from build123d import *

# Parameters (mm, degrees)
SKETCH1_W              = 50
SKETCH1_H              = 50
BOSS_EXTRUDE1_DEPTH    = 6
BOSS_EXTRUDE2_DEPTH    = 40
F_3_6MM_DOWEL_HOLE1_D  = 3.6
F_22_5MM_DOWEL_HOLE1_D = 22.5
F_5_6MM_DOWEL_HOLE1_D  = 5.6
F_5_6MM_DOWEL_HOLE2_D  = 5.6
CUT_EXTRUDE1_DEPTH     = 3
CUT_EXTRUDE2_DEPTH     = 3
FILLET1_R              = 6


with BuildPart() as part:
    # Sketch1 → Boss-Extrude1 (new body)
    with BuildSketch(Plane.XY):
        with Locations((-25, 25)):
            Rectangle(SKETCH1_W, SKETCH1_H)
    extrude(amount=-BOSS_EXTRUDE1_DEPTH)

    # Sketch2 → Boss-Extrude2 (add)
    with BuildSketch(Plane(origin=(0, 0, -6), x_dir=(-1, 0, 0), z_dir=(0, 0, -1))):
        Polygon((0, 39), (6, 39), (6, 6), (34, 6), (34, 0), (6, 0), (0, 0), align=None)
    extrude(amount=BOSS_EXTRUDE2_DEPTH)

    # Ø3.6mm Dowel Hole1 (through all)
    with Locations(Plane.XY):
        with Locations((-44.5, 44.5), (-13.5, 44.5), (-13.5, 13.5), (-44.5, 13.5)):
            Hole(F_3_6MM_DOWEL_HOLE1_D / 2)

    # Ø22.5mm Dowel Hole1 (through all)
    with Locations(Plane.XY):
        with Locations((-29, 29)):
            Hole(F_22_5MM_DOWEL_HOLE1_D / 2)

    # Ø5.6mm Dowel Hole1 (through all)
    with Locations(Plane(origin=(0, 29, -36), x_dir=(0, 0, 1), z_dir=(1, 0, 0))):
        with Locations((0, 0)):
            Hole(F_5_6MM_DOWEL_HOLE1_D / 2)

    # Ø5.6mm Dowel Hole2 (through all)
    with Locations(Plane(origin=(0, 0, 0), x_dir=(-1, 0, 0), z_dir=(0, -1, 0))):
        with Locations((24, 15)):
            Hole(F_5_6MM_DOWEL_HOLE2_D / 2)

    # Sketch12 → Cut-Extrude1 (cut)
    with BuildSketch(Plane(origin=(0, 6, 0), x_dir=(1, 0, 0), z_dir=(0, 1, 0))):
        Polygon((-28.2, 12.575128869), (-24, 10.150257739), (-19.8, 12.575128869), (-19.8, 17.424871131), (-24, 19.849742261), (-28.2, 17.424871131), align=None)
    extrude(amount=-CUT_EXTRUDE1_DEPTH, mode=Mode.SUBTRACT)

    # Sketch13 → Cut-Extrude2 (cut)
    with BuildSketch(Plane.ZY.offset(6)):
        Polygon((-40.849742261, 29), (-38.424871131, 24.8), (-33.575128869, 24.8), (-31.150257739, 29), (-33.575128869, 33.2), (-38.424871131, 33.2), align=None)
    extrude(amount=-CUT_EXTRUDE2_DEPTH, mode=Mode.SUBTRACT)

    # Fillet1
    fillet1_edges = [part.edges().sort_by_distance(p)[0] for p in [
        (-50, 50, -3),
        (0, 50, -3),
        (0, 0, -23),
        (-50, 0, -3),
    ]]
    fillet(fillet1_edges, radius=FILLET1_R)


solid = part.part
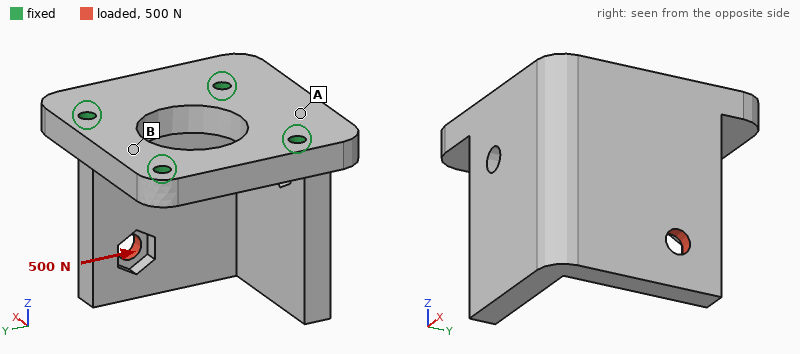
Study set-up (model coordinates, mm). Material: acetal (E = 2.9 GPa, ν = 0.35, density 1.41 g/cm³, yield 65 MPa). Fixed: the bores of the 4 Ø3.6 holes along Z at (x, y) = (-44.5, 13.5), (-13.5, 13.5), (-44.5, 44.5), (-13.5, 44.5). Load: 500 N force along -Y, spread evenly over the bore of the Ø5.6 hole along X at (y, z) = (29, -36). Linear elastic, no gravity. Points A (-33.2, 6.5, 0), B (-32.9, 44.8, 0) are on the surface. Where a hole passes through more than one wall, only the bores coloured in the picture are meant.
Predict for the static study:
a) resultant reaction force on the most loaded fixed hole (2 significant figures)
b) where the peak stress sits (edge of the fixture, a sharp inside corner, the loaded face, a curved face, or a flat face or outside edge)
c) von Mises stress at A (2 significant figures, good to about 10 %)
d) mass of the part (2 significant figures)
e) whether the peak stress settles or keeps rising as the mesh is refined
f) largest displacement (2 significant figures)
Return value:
590 N
edge of the fixture
7.2 MPa
39 g
keeps rising
0.84 mm
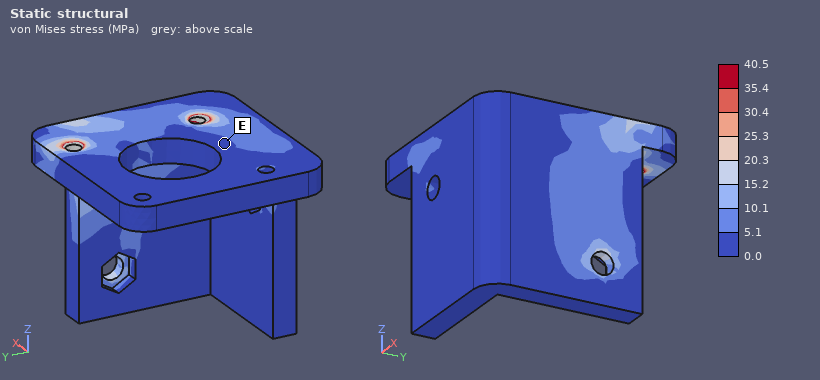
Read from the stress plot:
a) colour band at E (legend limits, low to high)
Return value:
0.0 to 5.1 MPa
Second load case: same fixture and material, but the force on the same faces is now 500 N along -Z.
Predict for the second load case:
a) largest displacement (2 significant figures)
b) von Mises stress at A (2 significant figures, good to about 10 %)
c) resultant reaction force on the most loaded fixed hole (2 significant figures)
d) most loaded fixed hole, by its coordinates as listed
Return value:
0.65 mm
4.6 MPa
330 N
(-13.5, 13.5)
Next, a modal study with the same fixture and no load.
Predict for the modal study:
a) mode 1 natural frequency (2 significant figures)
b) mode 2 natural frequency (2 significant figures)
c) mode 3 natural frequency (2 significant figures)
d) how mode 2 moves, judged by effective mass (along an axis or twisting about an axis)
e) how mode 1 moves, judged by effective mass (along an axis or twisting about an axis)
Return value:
910 Hz
1000 Hz
2000 Hz
along Y
along X
